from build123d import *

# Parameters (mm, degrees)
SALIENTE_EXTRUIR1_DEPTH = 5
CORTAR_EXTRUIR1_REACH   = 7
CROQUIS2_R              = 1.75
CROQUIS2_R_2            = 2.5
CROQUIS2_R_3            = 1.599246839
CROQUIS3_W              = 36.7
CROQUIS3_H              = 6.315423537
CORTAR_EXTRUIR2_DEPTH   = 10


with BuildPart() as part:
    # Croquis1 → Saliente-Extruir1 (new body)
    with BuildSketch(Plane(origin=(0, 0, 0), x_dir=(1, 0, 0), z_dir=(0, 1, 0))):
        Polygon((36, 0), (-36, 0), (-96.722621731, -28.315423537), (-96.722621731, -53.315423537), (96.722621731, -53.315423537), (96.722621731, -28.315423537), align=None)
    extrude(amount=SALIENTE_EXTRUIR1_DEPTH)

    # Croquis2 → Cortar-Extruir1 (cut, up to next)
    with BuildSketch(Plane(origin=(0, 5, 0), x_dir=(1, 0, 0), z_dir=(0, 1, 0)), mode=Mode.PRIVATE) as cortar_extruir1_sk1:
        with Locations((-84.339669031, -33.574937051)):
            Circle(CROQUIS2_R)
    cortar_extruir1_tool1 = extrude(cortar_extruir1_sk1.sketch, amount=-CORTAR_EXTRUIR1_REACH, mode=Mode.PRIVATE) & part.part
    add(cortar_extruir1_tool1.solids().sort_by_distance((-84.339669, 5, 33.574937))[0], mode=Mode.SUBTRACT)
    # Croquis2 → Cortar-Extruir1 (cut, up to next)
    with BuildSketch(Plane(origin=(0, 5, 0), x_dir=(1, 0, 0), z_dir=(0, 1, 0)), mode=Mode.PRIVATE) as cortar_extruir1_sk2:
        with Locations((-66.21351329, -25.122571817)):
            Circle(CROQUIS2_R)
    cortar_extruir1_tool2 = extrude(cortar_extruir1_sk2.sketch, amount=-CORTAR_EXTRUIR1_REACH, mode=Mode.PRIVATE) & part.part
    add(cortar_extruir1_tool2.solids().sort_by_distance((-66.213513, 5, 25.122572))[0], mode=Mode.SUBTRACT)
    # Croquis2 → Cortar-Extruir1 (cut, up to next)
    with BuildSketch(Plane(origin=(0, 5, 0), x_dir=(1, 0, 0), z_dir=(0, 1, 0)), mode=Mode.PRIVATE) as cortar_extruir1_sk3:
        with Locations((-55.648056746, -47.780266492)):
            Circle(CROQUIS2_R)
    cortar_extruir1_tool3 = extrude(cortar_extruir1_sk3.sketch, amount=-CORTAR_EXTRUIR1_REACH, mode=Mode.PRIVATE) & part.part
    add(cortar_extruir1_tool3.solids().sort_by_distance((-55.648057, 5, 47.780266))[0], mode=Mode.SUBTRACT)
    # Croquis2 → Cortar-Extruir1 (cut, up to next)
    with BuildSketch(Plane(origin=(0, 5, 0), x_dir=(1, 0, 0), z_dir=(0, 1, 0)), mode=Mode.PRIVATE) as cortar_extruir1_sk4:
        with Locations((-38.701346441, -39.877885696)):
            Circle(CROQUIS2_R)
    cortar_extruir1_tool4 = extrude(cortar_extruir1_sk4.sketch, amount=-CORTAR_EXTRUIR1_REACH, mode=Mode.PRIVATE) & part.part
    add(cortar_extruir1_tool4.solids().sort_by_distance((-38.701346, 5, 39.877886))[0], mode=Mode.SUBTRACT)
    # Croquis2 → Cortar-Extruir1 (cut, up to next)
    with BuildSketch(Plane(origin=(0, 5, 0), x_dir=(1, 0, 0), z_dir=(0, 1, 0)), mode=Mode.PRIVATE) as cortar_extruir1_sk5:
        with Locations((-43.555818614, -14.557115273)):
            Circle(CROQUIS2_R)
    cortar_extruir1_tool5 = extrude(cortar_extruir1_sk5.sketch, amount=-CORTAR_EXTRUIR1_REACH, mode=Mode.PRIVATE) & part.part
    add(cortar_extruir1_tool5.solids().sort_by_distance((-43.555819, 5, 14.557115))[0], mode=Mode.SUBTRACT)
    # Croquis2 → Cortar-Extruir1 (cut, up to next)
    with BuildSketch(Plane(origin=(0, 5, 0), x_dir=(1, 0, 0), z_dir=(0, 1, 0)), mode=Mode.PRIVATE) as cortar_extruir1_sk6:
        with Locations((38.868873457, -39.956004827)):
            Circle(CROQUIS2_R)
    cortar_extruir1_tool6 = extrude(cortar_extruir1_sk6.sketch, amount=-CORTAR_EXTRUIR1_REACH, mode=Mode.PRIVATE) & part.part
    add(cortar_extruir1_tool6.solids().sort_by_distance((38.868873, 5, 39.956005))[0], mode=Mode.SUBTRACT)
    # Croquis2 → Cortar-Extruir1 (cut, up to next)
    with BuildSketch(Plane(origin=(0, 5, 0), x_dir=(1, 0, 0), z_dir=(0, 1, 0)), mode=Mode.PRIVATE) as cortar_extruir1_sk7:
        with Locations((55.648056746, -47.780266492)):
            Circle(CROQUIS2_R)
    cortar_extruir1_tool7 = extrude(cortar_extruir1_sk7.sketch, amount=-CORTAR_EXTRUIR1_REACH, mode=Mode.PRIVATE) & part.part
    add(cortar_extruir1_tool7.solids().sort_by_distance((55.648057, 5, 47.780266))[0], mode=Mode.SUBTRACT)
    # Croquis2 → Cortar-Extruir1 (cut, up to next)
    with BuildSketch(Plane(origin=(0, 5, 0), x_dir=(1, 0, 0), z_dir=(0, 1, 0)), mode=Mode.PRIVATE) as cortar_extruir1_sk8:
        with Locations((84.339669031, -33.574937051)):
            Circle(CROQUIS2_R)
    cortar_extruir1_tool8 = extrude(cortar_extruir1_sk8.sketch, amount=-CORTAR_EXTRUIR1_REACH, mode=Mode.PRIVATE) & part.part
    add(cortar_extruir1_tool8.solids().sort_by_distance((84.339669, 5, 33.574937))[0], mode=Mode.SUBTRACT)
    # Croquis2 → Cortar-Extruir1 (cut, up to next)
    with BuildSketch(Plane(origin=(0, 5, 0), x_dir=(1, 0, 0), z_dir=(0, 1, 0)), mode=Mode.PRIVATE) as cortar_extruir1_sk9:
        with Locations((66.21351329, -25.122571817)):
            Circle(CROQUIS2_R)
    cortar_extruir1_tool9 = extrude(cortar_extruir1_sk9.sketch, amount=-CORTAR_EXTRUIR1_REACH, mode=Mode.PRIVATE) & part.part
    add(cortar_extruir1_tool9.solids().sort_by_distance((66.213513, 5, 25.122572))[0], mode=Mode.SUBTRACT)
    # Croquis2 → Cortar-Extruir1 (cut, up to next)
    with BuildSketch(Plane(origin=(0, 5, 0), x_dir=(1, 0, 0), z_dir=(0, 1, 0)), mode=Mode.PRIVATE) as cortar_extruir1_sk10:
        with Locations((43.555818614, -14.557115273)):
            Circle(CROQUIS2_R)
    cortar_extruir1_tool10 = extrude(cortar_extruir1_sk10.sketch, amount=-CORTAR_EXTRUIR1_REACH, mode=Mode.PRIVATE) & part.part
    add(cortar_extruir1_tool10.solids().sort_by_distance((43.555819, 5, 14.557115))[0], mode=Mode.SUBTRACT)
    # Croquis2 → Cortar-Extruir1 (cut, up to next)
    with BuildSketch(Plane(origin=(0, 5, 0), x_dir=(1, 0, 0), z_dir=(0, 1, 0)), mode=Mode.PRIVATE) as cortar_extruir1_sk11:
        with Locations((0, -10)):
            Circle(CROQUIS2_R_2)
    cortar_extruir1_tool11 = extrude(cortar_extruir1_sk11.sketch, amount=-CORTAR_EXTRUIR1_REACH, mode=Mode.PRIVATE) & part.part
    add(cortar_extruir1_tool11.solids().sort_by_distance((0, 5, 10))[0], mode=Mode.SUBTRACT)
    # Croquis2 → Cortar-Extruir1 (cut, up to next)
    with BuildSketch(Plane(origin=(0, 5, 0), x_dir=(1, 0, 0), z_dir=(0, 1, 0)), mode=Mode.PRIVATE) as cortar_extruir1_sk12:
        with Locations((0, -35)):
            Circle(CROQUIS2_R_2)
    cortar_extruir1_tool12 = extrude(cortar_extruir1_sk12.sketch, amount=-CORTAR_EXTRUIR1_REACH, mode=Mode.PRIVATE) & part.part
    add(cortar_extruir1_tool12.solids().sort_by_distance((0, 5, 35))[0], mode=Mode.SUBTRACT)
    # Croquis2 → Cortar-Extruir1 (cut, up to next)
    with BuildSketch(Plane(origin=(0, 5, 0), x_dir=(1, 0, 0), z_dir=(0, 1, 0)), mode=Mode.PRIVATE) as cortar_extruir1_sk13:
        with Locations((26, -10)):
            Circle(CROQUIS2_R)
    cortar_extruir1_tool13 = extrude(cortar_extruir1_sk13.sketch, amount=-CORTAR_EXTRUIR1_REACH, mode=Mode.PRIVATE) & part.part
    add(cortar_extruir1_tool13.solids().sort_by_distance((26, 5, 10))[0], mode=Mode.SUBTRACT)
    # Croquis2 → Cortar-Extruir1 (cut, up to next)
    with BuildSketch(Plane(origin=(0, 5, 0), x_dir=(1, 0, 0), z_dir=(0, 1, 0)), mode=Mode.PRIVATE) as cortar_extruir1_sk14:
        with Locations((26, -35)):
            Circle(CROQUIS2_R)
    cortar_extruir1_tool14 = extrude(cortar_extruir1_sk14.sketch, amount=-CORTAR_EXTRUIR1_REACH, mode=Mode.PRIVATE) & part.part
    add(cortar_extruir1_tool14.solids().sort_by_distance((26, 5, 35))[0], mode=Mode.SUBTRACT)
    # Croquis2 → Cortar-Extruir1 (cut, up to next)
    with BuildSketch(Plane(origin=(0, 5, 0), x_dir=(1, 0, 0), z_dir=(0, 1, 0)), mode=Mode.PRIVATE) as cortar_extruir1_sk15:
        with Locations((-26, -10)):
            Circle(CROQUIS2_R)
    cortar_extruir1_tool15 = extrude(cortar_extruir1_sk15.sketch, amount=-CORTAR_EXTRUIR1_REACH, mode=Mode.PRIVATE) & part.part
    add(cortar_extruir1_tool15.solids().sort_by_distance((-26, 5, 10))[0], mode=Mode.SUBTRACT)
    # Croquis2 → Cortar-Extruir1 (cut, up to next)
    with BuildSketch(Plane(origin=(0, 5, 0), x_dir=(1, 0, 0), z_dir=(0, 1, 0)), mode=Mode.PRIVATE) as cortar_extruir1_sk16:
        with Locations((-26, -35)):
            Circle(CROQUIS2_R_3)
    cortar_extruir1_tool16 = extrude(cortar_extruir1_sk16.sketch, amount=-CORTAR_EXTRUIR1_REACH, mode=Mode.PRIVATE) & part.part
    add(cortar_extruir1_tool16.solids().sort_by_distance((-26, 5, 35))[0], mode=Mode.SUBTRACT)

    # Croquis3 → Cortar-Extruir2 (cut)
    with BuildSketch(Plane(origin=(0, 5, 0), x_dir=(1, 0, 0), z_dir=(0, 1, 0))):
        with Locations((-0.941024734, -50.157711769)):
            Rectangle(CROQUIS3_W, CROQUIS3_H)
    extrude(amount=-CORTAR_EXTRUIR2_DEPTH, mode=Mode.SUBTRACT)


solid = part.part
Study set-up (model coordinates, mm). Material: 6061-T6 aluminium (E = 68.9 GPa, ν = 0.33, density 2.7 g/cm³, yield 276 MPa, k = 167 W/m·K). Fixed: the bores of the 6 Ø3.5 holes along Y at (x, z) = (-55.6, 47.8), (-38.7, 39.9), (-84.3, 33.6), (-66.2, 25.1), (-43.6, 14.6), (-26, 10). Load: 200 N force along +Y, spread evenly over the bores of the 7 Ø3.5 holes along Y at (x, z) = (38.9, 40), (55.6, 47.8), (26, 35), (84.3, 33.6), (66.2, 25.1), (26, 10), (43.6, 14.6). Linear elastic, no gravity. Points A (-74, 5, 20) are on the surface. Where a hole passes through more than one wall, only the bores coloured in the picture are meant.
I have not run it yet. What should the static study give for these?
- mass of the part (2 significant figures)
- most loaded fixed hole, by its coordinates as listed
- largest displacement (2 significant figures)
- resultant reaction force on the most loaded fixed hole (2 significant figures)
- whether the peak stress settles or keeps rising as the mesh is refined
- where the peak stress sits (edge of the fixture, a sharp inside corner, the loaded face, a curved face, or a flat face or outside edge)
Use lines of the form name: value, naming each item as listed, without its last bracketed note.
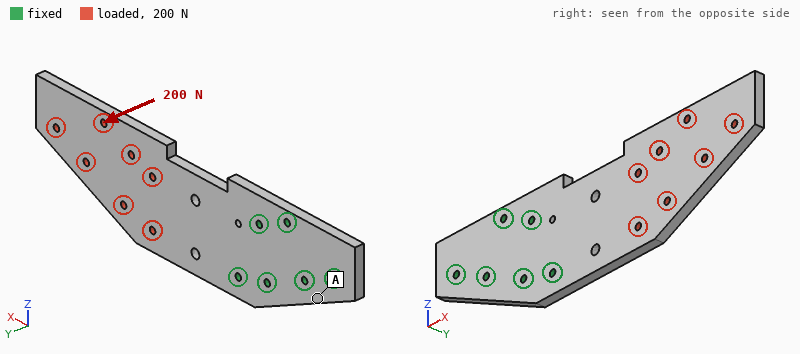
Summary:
mass of the part: 110 g
most loaded fixed hole, by its coordinates as listed: (-26, 10)
largest displacement: 2.0 mm
resultant reaction force on the most loaded fixed hole: 440 N
whether the peak stress settles or keeps rising as the mesh is refined: keeps rising
where the peak stress sits: edge of the fixture
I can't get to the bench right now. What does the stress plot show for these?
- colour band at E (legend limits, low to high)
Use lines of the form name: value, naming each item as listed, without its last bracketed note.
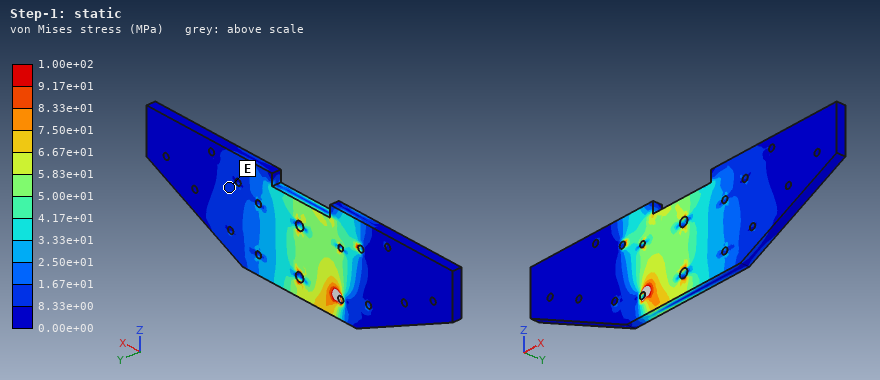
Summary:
colour band at E: 8.33e+00 to 1.67e+01 MPa
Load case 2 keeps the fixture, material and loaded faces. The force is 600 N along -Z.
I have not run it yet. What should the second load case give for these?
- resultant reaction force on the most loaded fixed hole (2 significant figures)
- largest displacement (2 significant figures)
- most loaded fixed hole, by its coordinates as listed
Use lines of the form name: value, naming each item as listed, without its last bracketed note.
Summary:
resultant reaction force on the most loaded fixed hole: 1.3 kN
largest displacement: 86 µm
most loaded fixed hole, by its coordinates as listed: (-26, 10)
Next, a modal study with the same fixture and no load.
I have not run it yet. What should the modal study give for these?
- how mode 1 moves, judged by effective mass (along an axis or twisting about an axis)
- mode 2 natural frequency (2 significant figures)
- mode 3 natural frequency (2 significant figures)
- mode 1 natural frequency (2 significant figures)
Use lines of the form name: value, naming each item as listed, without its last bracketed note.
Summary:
how mode 1 moves, judged by effective mass: along Y
mode 2 natural frequency: 1500 Hz
mode 3 natural frequency: 1700 Hz
mode 1 natural frequency: 290 Hz
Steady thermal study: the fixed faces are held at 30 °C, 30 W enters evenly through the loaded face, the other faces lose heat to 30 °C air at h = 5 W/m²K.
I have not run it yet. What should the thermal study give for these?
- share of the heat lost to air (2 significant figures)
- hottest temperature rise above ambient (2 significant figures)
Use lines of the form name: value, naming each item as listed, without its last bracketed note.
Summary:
share of the heat lost to air: 8.2 %
hottest temperature rise above ambient: 61 K
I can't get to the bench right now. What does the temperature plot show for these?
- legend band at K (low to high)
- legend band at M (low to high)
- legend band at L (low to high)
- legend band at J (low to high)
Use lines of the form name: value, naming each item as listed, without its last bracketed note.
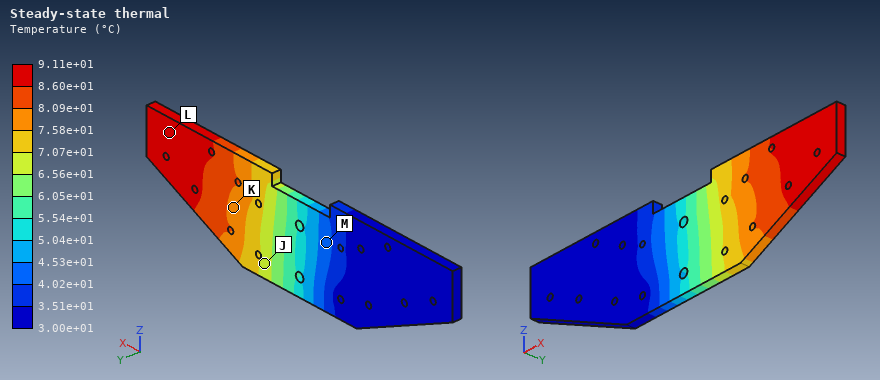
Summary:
legend band at K: 7.58e+01 to 8.09e+01 °C
legend band at M: 4.02e+01 to 4.53e+01 °C
legend band at L: 8.60e+01 to 9.11e+01 °C
legend band at J: 6.56e+01 to 7.07e+01 °C
